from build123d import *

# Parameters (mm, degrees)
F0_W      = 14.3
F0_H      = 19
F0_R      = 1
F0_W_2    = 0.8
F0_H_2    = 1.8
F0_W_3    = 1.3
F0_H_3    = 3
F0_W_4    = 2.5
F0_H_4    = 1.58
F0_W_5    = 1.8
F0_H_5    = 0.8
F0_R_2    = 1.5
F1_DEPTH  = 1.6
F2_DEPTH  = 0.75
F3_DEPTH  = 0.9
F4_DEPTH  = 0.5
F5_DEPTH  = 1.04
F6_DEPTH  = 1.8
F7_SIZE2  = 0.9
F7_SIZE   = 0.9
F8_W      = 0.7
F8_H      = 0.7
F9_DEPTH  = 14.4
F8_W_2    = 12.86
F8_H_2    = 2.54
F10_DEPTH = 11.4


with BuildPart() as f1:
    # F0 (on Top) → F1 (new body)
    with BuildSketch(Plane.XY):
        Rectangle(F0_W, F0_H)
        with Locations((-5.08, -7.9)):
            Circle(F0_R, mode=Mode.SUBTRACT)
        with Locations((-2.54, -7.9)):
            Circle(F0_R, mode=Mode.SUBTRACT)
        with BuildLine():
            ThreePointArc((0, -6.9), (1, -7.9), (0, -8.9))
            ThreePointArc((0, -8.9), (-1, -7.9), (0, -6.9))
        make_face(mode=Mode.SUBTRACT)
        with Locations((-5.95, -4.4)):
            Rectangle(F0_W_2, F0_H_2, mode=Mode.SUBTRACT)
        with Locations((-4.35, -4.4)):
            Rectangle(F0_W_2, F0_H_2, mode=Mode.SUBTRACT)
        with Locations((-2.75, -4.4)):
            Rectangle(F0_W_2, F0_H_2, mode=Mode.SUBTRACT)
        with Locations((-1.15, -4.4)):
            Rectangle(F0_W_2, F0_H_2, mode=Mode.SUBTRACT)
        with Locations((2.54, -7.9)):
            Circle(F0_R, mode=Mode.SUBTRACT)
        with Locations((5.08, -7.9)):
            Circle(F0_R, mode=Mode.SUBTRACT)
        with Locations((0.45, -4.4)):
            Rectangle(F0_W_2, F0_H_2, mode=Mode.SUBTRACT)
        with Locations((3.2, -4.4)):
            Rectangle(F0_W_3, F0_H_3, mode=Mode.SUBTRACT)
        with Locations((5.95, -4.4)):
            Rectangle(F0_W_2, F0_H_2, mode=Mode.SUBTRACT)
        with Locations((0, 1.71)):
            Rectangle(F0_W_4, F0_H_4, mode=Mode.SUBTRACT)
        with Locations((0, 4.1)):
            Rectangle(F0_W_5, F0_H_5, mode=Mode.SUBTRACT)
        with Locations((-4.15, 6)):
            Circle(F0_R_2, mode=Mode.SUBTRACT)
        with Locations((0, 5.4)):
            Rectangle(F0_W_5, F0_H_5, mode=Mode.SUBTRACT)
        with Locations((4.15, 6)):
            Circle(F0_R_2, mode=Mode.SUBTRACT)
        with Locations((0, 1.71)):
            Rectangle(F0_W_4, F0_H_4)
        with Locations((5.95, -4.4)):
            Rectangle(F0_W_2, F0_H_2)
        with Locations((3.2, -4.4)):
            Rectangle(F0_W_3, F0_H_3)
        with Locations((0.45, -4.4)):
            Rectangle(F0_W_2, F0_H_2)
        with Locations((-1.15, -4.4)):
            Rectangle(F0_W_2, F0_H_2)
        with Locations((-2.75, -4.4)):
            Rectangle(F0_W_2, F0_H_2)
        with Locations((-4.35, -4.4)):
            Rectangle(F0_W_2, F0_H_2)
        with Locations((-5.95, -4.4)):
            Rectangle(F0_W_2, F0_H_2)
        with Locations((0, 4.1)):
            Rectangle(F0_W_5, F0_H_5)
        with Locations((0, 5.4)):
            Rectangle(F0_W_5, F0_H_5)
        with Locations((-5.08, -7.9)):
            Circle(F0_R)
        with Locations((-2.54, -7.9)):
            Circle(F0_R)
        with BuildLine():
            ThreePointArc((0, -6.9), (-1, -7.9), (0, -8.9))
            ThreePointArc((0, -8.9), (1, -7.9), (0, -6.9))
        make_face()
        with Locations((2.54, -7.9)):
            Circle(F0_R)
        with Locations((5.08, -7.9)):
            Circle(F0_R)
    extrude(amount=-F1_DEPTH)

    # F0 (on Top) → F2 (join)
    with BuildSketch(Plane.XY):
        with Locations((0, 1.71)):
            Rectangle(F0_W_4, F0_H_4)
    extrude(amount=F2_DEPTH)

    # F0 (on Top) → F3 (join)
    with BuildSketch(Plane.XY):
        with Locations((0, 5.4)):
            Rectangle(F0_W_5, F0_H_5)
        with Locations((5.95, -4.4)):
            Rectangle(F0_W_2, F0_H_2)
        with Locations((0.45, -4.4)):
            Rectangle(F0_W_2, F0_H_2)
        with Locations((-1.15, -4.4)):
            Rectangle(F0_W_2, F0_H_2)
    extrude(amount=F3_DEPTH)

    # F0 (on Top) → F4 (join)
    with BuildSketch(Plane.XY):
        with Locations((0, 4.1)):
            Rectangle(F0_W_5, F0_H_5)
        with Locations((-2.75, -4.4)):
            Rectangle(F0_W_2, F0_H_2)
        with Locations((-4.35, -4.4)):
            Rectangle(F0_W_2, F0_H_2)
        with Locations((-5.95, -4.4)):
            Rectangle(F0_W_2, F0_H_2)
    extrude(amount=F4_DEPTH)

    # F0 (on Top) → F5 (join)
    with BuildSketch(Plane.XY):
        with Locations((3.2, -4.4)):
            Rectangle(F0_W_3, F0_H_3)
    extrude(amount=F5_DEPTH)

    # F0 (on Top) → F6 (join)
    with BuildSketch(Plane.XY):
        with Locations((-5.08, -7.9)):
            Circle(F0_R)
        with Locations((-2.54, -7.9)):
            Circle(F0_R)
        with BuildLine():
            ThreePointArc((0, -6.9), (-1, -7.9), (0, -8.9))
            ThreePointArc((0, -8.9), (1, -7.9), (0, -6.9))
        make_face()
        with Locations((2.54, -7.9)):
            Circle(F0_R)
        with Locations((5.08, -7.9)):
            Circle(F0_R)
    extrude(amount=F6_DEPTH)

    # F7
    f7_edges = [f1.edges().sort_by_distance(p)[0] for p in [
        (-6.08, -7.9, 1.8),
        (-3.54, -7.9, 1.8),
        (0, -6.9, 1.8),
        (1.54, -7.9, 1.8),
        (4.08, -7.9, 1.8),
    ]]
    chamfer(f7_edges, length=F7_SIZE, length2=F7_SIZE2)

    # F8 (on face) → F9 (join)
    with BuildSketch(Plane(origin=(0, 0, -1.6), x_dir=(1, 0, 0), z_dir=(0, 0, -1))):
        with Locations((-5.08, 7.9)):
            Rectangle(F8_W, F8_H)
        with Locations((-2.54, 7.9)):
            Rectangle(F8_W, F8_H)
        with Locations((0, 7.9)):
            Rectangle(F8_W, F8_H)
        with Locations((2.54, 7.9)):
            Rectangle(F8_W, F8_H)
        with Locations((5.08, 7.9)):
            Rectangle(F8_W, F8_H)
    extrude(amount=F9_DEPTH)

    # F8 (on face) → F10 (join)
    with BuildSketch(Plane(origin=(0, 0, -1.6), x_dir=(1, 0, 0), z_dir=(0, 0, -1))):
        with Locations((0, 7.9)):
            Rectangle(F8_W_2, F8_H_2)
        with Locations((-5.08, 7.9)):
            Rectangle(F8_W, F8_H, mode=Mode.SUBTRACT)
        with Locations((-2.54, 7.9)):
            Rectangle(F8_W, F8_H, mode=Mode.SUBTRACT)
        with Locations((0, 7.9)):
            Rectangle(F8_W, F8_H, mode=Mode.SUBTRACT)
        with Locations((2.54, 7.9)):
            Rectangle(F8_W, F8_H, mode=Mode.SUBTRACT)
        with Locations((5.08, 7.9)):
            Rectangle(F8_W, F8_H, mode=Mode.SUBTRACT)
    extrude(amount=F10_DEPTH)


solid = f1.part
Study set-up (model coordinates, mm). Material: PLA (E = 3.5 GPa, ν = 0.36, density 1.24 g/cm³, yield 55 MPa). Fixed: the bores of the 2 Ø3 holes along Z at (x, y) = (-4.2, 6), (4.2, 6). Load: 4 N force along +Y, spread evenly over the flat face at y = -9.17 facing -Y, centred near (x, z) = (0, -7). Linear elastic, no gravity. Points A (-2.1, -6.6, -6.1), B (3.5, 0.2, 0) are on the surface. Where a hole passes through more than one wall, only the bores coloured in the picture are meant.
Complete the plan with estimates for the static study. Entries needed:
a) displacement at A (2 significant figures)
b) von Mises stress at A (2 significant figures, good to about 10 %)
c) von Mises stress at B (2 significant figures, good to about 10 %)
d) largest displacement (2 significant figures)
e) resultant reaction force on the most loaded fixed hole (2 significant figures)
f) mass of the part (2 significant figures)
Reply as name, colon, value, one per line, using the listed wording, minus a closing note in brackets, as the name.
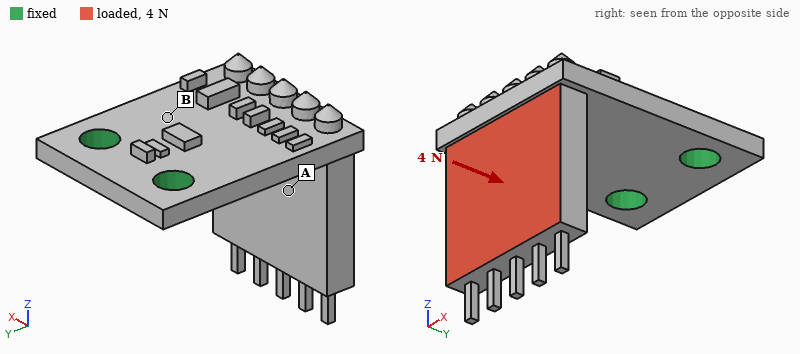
displacement at A: 0.13 mm
von Mises stress at A: 0.61 MPa
von Mises stress at B: 3.7 MPa
largest displacement: 0.30 mm
resultant reaction force on the most loaded fixed hole: 2.0 N
mass of the part: 1.0 g
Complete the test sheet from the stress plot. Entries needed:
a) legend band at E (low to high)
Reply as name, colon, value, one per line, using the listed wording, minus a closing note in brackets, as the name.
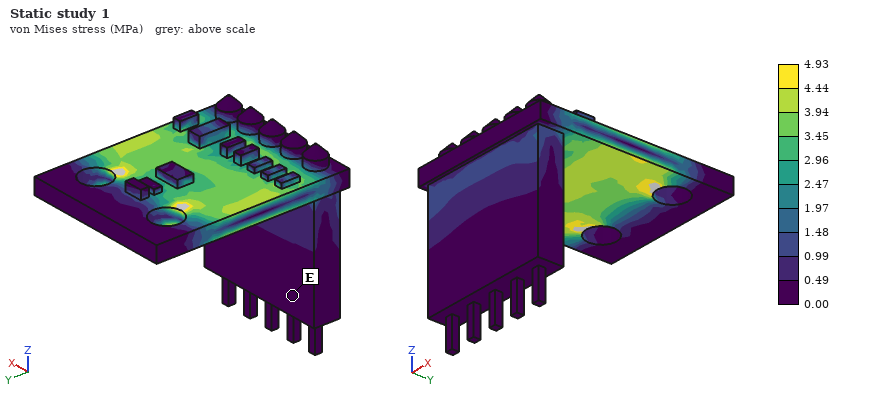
legend band at E: 0.00 to 0.49 MPa
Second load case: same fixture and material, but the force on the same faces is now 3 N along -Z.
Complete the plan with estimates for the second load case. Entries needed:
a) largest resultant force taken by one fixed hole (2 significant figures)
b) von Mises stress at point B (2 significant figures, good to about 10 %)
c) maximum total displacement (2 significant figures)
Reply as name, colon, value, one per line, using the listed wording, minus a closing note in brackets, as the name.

largest resultant force taken by one fixed hole: 1.5 N
von Mises stress at point B: 4.1 MPa
maximum total displacement: 0.28 mm
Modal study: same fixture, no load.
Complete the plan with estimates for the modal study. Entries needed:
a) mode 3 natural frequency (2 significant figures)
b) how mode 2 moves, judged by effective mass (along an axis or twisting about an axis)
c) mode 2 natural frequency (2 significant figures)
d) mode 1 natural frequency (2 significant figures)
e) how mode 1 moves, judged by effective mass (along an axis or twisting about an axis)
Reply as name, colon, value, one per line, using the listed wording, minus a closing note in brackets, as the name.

mode 3 natural frequency: 2800 Hz
how mode 2 moves, judged by effective mass: along X
mode 2 natural frequency: 1600 Hz
mode 1 natural frequency: 800 Hz
how mode 1 moves, judged by effective mass: along Z
